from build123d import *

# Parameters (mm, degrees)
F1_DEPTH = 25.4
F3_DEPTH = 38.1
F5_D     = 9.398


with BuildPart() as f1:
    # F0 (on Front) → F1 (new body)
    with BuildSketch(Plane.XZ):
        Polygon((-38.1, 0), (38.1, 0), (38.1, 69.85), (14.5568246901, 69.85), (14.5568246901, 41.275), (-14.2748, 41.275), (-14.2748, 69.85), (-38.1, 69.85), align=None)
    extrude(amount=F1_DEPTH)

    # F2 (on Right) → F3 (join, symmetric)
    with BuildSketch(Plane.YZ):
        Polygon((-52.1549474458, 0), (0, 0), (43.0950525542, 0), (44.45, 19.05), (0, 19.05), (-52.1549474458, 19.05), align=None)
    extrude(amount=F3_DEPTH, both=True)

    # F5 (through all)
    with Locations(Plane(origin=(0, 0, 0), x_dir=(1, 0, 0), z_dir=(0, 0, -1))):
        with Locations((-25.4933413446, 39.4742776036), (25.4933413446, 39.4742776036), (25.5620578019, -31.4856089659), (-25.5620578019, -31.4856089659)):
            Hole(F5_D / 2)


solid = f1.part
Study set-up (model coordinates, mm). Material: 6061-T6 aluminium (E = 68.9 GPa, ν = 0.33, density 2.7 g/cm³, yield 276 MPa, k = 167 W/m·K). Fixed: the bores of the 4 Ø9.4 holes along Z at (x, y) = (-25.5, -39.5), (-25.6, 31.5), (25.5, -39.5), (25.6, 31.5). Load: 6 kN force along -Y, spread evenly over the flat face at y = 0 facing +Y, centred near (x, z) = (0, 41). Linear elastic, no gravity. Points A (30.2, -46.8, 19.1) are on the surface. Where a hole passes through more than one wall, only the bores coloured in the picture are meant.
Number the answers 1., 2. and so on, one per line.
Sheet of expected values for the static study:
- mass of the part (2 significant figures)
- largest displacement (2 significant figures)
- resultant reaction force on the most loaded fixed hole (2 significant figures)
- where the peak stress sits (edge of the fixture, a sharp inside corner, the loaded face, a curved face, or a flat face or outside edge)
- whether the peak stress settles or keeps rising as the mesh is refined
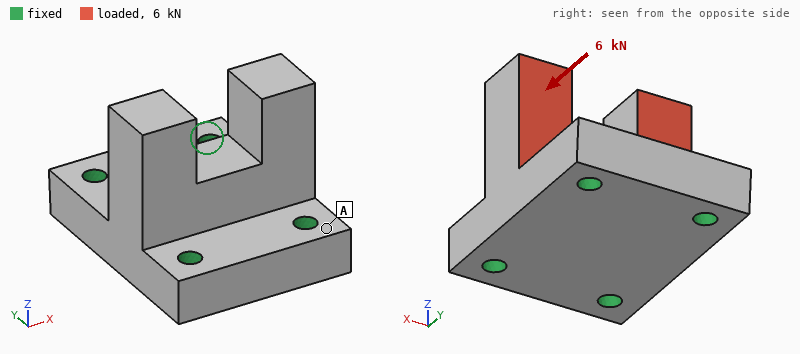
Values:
1. 570 g
2. 37 µm
3. 2.4 kN
4. edge of the fixture
5. keeps rising
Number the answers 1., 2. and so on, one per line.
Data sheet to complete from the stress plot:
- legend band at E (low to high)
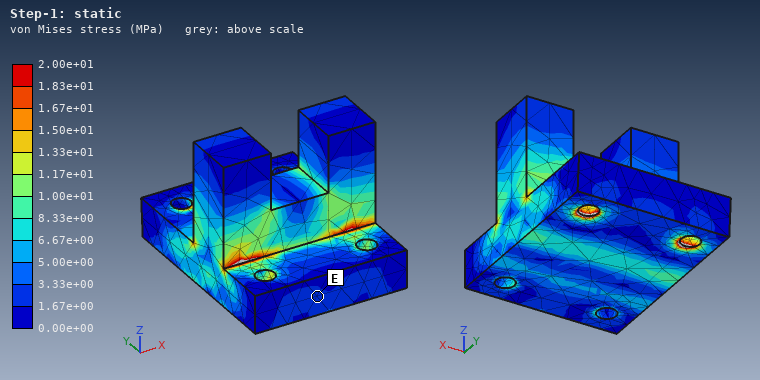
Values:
1. 1.67e+00 to 3.33e+00 MPa
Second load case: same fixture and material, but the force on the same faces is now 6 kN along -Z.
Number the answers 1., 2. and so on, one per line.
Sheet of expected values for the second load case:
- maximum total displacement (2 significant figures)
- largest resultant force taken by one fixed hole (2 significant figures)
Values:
1. 26 µm
2. 1.8 kN
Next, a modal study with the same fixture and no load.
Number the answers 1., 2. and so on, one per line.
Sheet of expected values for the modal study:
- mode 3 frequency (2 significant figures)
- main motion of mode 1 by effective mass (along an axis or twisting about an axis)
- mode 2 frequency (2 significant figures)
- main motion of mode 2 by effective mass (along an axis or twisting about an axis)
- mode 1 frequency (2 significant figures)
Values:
1. 6700 Hz
2. along Y
3. 5900 Hz
4. along X
5. 5500 Hz
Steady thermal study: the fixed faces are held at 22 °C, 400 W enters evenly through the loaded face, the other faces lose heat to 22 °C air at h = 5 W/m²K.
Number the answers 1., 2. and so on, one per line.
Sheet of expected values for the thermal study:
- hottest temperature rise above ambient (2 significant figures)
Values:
1. 69 K
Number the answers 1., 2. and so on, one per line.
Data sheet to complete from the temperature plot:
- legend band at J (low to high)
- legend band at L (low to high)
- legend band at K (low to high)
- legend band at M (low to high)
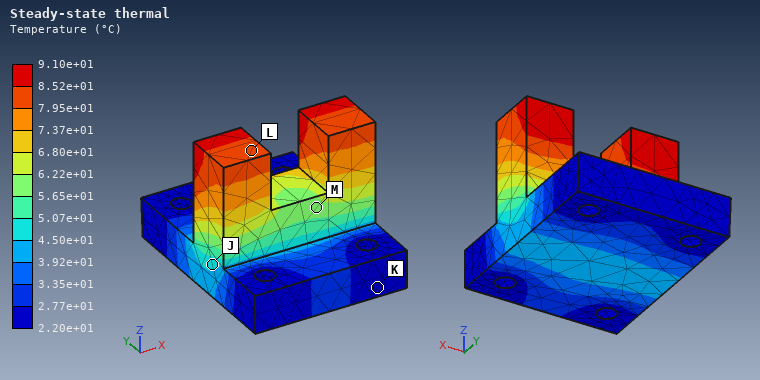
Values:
1. 4.50e+01 to 5.07e+01 °C
2. 7.95e+01 to 8.52e+01 °C
3. 2.20e+01 to 2.77e+01 °C
4. 5.65e+01 to 6.22e+01 °C
